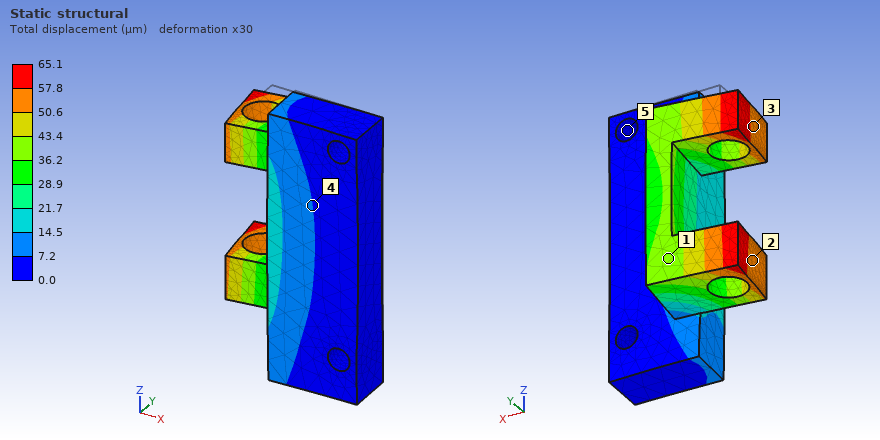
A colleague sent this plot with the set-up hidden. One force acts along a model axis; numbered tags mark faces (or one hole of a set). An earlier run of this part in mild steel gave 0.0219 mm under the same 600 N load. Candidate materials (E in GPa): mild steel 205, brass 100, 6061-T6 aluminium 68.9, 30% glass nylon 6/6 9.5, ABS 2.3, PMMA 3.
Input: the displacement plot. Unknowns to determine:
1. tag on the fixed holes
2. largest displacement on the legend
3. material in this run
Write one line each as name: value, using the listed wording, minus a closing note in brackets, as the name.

tag on the fixed holes: 5
largest displacement on the legend: 65.1 µm
material in this run: 6061-T6 aluminium
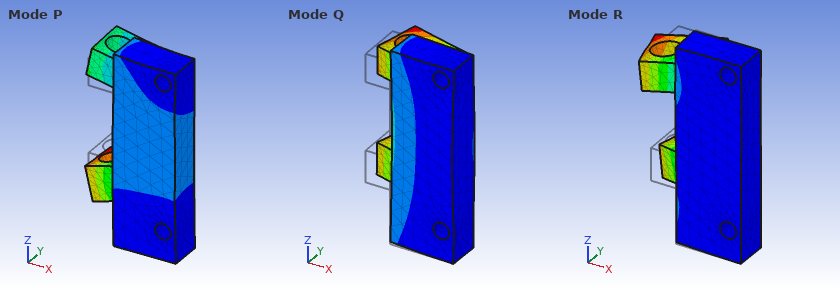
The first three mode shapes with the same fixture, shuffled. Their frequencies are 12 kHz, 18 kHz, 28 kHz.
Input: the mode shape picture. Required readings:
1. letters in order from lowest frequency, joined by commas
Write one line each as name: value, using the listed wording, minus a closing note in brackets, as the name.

letters in order from lowest frequency, joined by commas: Q, R, P
